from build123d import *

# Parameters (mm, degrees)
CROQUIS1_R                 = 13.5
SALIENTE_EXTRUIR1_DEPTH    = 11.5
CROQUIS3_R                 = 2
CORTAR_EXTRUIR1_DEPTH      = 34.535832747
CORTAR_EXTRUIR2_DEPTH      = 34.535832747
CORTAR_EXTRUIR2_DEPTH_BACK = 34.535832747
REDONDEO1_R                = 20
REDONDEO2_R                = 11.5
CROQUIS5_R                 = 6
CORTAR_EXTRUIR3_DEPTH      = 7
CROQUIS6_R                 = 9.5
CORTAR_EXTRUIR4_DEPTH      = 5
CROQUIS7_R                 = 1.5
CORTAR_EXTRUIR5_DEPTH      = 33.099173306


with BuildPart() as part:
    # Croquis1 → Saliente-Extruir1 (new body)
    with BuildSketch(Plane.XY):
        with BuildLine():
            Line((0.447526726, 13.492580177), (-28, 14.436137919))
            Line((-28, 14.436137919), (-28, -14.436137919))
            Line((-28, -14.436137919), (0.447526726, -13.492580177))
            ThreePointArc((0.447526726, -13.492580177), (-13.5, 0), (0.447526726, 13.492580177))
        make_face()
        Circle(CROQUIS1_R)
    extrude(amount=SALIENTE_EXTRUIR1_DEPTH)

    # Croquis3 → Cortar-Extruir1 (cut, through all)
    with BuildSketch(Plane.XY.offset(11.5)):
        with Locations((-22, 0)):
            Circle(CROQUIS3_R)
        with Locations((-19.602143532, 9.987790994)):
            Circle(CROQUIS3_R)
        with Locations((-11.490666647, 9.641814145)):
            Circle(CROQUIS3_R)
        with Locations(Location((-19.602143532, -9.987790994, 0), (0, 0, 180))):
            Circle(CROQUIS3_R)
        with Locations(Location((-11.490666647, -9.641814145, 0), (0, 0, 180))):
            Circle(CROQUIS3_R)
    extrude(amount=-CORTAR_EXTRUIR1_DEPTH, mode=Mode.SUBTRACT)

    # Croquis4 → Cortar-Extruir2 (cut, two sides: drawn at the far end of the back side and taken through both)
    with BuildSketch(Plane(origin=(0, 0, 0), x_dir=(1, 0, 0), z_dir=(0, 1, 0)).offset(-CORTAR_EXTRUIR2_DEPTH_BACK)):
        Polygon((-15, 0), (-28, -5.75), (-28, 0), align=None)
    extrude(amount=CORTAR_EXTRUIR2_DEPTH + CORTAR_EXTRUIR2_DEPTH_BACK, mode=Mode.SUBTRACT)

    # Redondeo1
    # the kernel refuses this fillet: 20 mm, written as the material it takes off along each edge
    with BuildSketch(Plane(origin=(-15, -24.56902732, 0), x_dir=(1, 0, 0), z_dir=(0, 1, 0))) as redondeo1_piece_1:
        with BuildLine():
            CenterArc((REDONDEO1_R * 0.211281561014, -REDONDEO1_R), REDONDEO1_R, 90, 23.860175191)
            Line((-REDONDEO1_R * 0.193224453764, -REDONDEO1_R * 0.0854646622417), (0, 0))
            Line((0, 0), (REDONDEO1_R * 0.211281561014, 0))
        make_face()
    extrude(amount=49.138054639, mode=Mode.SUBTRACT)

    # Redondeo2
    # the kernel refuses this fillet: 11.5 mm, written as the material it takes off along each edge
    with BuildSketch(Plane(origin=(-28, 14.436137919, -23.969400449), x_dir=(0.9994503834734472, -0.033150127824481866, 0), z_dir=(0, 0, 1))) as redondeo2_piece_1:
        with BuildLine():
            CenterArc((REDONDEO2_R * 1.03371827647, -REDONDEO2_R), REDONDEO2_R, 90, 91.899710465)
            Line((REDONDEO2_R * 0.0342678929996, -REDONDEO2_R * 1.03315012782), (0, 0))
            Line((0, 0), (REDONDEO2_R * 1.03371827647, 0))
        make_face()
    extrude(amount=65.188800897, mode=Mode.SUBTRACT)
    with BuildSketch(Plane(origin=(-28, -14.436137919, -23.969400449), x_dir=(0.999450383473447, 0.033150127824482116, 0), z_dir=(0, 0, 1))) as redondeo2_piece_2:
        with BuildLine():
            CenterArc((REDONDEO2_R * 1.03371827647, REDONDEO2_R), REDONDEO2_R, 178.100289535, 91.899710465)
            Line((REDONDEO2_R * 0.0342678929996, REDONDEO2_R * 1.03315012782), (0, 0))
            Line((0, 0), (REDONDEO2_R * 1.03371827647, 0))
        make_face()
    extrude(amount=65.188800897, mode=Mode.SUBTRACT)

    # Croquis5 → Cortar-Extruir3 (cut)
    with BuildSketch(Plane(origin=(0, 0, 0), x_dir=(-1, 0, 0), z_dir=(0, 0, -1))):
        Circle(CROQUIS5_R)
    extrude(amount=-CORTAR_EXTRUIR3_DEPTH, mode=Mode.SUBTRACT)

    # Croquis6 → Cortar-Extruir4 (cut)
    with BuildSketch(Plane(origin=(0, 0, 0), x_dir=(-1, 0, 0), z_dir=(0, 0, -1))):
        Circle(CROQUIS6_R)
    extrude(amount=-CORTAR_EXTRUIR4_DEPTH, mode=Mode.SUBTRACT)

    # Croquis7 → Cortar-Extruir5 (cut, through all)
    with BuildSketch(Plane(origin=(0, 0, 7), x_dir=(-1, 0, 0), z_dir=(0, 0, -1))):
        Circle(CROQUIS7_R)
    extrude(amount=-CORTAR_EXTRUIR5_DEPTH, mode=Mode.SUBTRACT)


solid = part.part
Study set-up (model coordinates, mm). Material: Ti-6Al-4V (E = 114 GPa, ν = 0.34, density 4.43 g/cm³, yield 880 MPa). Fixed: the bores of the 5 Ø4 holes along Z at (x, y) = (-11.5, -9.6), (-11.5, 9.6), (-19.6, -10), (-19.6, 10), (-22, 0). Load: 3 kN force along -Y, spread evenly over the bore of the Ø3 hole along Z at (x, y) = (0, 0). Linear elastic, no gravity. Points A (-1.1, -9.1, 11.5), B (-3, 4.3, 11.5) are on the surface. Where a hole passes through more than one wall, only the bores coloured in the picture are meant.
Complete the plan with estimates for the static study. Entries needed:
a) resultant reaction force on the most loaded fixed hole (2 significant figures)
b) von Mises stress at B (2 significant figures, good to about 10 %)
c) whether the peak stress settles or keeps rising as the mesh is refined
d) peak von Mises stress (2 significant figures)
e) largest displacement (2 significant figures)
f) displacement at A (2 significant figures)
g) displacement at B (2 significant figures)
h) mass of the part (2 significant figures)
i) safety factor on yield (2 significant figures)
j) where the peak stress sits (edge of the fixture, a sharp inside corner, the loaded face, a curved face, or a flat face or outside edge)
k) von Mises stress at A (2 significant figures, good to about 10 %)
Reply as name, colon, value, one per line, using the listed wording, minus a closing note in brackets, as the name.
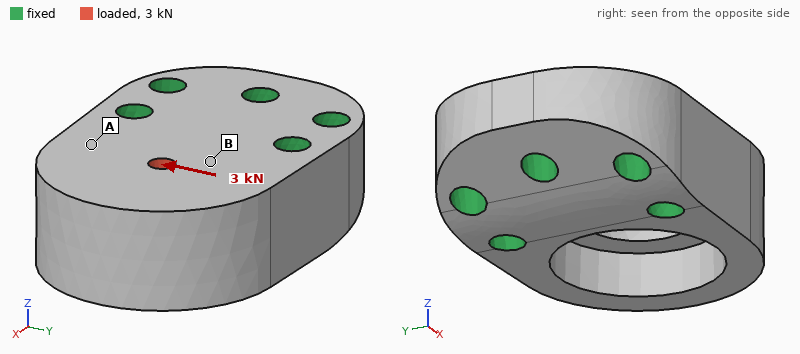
resultant reaction force on the most loaded fixed hole: 2.0 kN
von Mises stress at B: 48 MPa
whether the peak stress settles or keeps rising as the mesh is refined: settles
peak von Mises stress: 130 MPa
largest displacement: 8.4 µm
displacement at A: 5.0 µm
displacement at B: 4.2 µm
mass of the part: 37 g
safety factor on yield: 6.7
where the peak stress sits: the loaded face
von Mises stress at A: 22 MPa
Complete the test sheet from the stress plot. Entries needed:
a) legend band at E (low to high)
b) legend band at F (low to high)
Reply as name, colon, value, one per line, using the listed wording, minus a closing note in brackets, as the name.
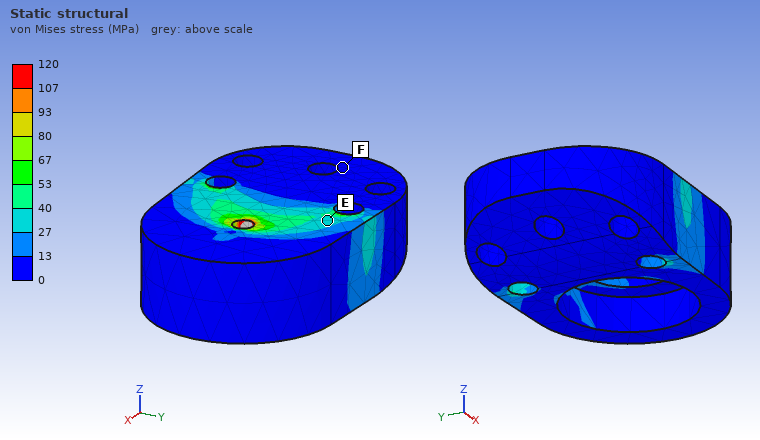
legend band at E: 27 to 40 MPa
legend band at F: 0 to 13 MPa
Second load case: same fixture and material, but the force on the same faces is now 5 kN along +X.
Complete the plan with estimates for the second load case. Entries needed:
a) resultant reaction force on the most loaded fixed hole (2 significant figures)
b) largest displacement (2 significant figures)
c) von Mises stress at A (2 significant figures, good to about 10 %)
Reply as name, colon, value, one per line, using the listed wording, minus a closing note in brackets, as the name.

resultant reaction force on the most loaded fixed hole: 1.9 kN
largest displacement: 12 µm
von Mises stress at A: 25 MPa
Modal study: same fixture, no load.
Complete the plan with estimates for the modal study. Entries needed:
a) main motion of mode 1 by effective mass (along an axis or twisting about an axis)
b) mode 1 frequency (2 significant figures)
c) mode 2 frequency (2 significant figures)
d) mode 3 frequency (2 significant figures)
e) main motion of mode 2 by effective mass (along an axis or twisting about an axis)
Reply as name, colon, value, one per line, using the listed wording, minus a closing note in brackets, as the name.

main motion of mode 1 by effective mass: along Z
mode 1 frequency: 13 kHz
mode 2 frequency: 21 kHz
mode 3 frequency: 30 kHz
main motion of mode 2 by effective mass: along Y
